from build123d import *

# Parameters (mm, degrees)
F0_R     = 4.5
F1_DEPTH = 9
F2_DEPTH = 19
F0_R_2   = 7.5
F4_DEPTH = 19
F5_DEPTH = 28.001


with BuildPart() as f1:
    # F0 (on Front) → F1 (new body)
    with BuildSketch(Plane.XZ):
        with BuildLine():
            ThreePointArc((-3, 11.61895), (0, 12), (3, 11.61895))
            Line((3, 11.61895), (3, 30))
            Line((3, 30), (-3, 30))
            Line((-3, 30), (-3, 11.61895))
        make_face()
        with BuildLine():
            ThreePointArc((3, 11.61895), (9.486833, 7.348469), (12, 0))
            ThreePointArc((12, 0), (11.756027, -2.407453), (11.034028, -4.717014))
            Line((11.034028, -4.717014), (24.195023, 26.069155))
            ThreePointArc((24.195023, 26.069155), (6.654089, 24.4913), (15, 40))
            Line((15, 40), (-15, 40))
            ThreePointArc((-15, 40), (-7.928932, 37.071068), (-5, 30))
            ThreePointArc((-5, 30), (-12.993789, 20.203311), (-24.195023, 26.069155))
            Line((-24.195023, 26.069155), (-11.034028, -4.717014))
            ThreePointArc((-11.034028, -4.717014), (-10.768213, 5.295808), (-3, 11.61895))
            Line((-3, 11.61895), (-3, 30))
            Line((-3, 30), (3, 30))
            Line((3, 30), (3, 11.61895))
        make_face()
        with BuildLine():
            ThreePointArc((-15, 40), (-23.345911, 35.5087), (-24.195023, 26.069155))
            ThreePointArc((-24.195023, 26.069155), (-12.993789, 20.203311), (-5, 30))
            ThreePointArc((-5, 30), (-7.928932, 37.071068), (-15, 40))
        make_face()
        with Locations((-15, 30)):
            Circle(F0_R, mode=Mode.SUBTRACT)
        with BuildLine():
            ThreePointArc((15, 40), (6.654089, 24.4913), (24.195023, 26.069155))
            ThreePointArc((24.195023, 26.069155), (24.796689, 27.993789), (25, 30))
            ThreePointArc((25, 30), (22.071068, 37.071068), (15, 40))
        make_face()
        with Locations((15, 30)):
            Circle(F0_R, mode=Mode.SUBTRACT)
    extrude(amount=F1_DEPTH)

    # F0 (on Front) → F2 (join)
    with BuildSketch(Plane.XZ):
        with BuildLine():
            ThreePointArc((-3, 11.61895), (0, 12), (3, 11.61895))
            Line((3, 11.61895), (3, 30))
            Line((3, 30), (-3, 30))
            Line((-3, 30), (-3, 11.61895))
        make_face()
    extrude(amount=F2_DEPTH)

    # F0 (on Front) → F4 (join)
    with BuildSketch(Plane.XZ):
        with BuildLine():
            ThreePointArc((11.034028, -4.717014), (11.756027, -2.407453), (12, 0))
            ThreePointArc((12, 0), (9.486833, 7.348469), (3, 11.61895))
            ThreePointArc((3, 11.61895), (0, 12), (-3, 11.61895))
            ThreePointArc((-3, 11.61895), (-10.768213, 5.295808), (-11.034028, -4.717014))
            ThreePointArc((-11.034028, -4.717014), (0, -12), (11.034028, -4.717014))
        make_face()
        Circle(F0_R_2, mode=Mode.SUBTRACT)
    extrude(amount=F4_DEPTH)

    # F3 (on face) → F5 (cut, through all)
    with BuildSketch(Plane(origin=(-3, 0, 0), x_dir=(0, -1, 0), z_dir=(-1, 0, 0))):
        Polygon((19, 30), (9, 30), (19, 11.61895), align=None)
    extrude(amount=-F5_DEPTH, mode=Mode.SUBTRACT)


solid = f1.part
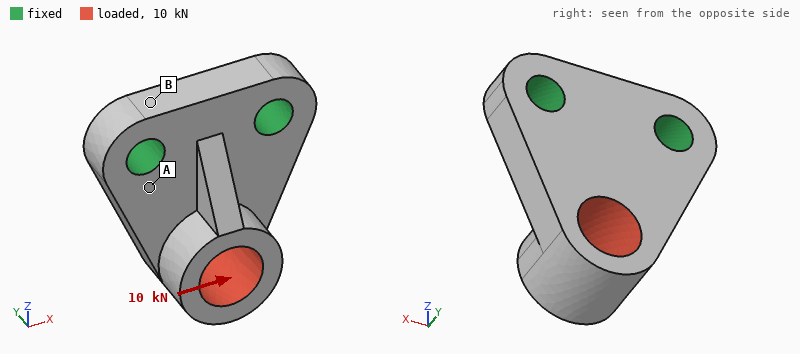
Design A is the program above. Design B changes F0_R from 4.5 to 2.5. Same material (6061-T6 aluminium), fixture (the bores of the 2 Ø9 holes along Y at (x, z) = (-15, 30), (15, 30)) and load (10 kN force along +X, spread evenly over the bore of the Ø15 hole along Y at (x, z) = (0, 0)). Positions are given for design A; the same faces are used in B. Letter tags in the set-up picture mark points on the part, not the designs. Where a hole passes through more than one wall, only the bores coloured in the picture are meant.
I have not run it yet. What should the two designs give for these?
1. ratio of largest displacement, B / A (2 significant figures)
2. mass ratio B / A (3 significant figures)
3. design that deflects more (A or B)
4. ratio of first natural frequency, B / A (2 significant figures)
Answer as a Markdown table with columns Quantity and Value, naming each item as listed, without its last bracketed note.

| Quantity | Value |
|---|---|
| ratio of largest displacement, B / A | 1.1 |
| mass ratio B / A | 1.05 |
| design that deflects more | B |
| ratio of first natural frequency, B / A | 0.86 |
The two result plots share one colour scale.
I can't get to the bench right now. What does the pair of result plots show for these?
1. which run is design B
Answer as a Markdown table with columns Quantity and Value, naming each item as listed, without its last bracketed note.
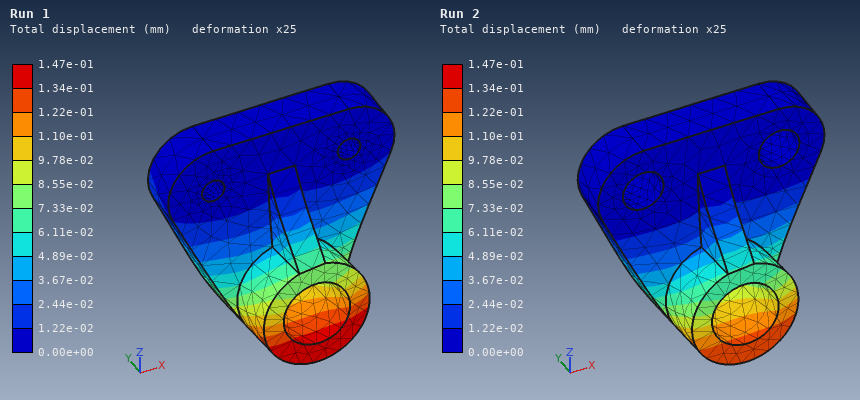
| Quantity | Value |
|---|---|
| which run is design B | Run 1 |
